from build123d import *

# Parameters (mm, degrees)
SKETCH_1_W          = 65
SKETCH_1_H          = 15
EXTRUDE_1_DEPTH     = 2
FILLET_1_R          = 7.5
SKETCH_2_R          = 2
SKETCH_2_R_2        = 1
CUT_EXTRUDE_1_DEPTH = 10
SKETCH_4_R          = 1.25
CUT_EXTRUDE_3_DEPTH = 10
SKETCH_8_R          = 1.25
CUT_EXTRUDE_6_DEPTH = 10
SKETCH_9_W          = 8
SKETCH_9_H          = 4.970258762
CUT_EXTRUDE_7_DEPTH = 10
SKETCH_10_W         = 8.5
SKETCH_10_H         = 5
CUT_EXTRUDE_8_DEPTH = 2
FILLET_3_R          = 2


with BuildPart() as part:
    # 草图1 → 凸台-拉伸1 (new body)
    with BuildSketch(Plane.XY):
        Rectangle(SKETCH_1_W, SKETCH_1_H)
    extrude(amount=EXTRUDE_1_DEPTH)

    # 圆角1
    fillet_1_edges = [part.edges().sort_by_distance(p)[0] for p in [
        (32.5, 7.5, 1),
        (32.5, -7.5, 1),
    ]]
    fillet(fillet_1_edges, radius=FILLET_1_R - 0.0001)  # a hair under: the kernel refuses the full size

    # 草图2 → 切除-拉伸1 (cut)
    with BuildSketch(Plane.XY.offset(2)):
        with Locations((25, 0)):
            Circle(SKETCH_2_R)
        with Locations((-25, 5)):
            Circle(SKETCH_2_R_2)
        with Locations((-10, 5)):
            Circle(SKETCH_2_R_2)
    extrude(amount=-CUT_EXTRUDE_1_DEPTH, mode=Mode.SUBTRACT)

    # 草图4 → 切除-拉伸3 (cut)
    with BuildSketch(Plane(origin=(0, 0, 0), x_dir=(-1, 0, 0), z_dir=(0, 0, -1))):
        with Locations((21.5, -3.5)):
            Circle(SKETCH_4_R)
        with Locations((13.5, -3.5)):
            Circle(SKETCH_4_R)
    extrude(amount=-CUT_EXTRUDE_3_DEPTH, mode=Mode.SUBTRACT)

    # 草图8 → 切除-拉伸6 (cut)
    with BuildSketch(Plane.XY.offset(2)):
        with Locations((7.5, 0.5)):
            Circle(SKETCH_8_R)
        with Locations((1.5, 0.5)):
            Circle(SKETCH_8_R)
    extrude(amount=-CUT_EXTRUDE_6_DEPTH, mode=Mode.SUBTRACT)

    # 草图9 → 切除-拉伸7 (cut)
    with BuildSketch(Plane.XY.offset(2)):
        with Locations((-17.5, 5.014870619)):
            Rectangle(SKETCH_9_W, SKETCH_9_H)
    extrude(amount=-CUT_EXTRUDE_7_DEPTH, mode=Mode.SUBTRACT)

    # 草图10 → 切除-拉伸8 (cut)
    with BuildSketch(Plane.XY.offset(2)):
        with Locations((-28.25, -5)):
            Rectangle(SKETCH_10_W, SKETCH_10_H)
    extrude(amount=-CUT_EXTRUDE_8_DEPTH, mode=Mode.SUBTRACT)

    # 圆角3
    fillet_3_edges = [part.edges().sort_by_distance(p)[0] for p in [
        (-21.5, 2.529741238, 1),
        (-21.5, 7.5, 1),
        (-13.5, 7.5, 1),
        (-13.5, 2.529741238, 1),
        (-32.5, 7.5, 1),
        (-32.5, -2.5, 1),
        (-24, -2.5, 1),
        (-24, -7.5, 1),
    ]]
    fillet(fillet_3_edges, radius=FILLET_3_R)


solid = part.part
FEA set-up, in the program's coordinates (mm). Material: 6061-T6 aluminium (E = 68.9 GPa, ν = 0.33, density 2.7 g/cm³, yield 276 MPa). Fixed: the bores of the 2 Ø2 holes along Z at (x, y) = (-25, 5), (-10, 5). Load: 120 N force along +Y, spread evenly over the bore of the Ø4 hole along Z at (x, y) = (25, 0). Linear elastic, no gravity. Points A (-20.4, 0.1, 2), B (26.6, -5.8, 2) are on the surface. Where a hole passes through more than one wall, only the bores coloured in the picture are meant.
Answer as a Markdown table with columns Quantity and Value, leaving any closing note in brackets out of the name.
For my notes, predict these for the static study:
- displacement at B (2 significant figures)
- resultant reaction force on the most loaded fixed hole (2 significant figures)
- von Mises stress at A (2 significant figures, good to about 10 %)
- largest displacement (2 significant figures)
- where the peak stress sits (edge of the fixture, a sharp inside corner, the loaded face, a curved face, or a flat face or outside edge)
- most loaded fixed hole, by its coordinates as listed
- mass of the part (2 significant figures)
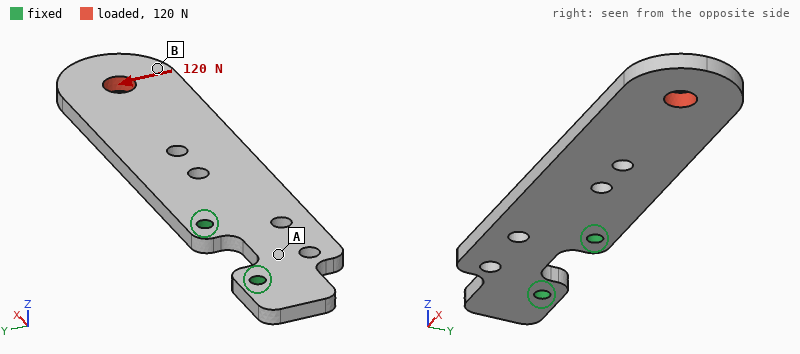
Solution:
| Quantity | Value |
|---|---|
| displacement at B | 0.094 mm |
| resultant reaction force on the most loaded fixed hole | 400 N |
| von Mises stress at A | 29 MPa |
| largest displacement | 0.11 mm |
| where the peak stress sits | edge of the fixture |
| most loaded fixed hole, by its coordinates as listed | (-10, 5) |
| mass of the part | 4.5 g |
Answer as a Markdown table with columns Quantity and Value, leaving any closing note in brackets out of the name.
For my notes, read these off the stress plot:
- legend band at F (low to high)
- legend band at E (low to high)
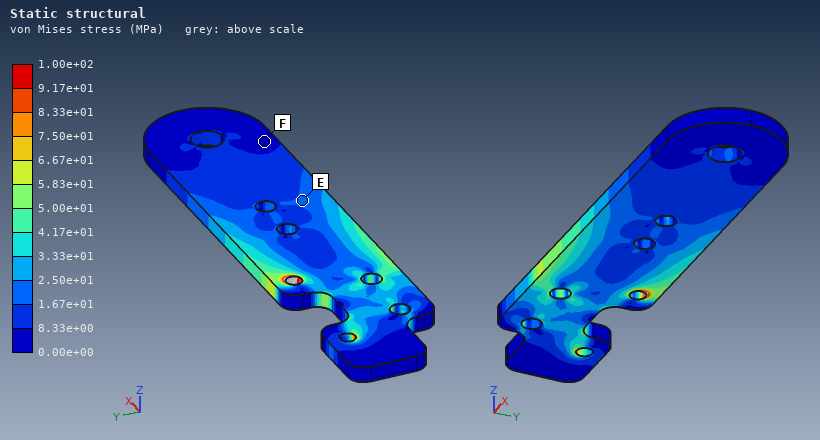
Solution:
| Quantity | Value |
|---|---|
| legend band at F | 0.00e+00 to 8.33e+00 MPa |
| legend band at E | 1.67e+01 to 2.50e+01 MPa |
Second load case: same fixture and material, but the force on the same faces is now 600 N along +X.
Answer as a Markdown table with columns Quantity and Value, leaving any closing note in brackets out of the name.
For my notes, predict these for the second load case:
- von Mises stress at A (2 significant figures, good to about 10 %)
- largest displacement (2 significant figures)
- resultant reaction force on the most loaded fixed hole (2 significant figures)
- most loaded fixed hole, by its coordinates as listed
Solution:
| Quantity | Value |
|---|---|
| von Mises stress at A | 21 MPa |
| largest displacement | 36 µm |
| resultant reaction force on the most loaded fixed hole | 450 N |
| most loaded fixed hole, by its coordinates as listed | (-10, 5) |
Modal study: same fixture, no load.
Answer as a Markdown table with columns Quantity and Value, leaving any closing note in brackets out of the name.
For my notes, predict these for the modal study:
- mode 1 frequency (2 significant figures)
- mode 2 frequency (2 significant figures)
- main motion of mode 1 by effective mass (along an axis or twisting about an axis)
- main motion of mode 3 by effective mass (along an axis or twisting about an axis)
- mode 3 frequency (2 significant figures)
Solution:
| Quantity | Value |
|---|---|
| mode 1 frequency | 920 Hz |
| mode 2 frequency | 4300 Hz |
| main motion of mode 1 by effective mass | along Z |
| main motion of mode 3 by effective mass | along Y |
| mode 3 frequency | 5000 Hz |
